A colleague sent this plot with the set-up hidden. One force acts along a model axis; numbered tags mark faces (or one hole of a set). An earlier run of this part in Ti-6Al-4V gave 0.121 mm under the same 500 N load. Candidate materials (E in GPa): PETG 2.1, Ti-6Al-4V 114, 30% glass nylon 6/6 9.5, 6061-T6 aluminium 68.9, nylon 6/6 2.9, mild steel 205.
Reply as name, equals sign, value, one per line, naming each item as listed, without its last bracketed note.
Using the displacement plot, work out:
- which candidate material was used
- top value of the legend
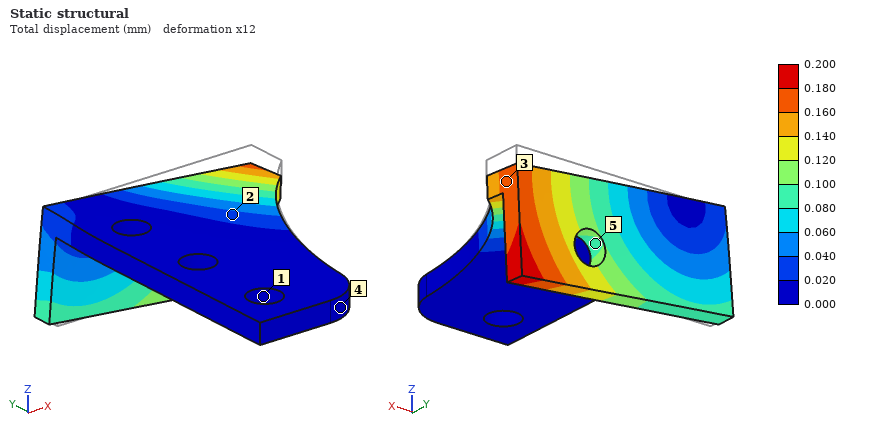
which candidate material was used = 6061-T6 aluminium
top value of the legend = 0.200 mm
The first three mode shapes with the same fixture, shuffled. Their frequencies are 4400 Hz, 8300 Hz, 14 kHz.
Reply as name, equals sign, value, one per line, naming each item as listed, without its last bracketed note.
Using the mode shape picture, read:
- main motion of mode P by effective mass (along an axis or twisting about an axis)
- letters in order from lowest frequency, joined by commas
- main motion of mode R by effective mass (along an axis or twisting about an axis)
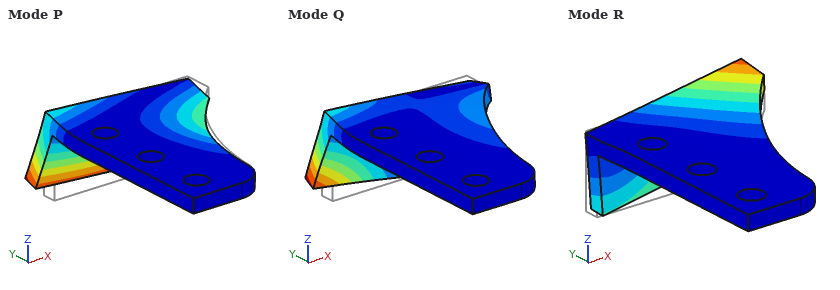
main motion of mode P by effective mass = along Y
letters in order from lowest frequency, joined by commas = R, P, Q
main motion of mode R by effective mass = along Z
